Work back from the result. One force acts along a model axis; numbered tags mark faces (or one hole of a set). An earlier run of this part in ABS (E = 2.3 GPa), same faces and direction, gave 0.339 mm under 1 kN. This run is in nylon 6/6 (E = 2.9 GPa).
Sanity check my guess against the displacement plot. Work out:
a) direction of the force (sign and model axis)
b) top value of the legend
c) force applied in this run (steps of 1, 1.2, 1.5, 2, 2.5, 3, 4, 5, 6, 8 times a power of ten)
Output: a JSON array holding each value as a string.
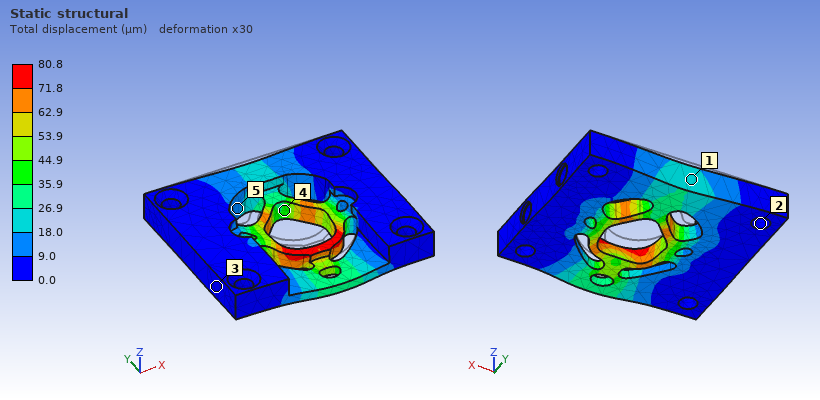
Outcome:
["-Y", "80.8 µm", "300 N"]
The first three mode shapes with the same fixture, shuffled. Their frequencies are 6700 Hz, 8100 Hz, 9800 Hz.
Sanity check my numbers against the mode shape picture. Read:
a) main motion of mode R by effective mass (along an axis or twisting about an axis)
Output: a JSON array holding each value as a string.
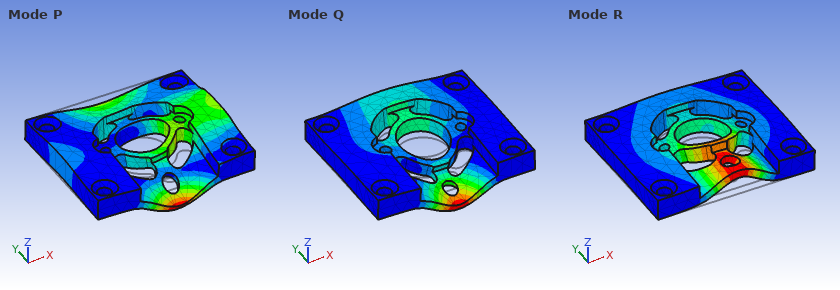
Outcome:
["along Z"]
